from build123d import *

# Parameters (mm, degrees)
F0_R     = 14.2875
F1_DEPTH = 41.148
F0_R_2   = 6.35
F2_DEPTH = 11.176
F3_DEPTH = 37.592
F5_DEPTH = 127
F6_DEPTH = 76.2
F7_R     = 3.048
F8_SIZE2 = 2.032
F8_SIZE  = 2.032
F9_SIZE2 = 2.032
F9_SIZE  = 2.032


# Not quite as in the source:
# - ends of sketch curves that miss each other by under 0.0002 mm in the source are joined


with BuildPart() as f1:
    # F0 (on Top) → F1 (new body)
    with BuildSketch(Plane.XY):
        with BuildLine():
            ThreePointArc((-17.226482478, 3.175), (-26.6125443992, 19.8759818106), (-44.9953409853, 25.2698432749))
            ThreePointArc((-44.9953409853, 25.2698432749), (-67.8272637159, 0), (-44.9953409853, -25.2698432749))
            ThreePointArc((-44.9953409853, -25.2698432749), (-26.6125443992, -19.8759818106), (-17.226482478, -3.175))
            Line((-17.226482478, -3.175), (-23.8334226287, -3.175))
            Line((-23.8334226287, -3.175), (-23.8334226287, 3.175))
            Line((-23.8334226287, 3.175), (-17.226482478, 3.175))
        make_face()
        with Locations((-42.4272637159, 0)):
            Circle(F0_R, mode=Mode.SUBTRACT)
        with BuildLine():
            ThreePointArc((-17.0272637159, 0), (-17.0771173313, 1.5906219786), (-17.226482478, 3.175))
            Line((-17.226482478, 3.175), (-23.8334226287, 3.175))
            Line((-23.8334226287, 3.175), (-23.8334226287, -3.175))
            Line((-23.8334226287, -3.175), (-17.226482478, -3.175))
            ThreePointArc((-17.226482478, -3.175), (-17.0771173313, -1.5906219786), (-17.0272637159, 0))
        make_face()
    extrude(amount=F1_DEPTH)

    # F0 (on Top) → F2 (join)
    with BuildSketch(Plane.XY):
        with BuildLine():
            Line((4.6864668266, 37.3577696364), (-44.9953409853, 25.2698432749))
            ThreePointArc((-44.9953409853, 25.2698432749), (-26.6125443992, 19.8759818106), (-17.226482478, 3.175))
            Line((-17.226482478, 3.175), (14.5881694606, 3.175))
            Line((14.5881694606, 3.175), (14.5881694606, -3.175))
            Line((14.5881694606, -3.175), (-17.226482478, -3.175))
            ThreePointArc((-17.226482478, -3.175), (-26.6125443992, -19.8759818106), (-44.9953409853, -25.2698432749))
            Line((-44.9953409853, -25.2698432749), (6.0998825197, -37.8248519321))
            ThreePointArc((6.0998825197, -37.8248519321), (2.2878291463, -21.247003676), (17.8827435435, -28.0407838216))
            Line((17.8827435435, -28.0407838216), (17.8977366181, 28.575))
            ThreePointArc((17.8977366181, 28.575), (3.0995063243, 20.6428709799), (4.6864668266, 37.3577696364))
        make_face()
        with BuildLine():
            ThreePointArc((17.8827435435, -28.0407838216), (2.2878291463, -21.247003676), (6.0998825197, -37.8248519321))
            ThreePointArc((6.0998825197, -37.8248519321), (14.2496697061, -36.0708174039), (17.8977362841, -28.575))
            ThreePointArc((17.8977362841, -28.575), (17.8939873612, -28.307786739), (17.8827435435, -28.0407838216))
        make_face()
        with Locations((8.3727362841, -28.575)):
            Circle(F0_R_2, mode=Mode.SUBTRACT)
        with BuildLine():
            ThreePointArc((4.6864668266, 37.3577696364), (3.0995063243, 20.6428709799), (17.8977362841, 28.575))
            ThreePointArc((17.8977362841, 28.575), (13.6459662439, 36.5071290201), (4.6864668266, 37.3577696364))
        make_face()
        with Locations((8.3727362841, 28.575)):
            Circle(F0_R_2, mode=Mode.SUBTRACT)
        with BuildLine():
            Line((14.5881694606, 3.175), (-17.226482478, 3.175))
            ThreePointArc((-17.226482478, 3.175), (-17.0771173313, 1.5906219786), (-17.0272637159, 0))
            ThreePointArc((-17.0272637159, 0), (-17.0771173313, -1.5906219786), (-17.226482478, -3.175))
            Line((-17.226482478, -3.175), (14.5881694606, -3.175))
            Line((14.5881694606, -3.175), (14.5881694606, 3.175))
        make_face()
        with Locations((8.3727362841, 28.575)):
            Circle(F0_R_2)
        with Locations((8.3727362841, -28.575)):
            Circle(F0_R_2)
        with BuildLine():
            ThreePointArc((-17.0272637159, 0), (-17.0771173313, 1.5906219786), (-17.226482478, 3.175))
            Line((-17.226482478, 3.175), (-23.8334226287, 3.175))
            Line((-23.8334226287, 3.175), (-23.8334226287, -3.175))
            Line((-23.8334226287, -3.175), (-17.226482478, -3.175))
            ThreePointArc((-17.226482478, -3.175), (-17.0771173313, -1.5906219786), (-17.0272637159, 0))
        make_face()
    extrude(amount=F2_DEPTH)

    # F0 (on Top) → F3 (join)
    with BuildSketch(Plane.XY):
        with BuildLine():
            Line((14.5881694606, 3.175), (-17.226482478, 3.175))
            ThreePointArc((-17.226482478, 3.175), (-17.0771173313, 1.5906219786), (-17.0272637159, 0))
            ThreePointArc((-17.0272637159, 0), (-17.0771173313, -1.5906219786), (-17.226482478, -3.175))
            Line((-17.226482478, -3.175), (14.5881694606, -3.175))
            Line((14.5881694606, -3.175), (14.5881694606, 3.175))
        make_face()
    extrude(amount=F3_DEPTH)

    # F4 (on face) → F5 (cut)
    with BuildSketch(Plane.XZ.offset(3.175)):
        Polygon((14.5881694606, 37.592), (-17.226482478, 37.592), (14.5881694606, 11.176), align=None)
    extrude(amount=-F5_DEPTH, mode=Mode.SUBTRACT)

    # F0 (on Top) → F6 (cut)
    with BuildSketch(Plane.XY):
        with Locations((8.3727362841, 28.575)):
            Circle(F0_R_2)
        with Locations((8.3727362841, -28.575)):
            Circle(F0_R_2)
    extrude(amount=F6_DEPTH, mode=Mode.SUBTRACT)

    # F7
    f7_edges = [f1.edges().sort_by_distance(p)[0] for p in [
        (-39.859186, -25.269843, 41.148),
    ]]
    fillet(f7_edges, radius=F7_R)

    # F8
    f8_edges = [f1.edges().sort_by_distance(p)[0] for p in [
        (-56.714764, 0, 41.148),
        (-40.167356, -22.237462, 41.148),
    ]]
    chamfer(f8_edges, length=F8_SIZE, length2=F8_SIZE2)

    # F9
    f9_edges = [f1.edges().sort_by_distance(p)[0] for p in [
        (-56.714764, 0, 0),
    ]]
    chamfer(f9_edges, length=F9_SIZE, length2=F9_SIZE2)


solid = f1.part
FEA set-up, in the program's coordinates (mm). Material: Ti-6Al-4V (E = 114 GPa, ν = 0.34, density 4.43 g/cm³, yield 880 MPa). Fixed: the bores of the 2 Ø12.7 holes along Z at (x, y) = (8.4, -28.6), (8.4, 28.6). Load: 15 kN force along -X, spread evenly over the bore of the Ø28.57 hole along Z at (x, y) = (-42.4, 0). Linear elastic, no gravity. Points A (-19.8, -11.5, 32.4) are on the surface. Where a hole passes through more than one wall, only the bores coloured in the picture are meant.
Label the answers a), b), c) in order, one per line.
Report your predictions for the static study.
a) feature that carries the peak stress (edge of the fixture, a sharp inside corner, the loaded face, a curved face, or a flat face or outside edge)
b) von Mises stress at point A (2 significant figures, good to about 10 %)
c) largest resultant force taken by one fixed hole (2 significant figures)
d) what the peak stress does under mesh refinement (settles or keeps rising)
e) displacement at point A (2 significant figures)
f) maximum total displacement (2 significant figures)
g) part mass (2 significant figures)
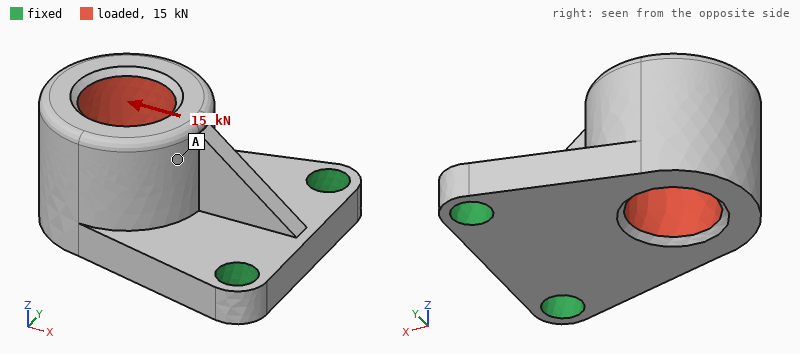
a) edge of the fixture
b) 25 MPa
c) 8.0 kN
d) keeps rising
e) 0.15 mm
f) 0.36 mm
g) 390 g
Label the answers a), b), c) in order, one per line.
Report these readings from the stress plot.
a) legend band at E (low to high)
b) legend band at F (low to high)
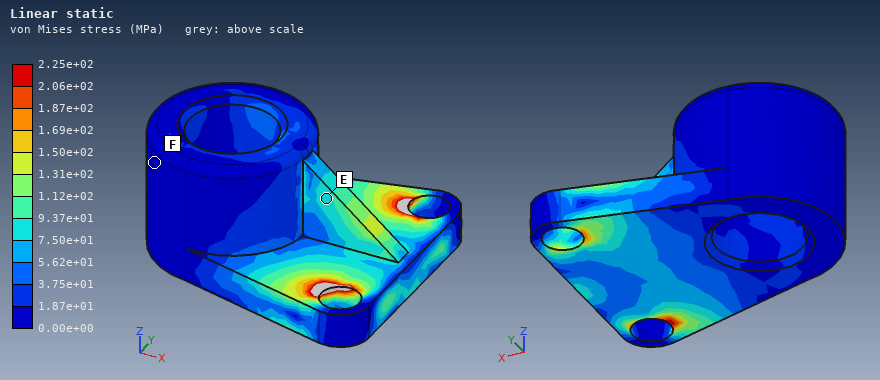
a) 7.50e+01 to 9.37e+01 MPa
b) 0.00e+00 to 1.87e+01 MPa
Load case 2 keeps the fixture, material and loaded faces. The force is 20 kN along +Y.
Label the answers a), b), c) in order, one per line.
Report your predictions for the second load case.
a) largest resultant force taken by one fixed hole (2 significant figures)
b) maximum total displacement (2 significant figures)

a) 20 kN
b) 0.19 mm
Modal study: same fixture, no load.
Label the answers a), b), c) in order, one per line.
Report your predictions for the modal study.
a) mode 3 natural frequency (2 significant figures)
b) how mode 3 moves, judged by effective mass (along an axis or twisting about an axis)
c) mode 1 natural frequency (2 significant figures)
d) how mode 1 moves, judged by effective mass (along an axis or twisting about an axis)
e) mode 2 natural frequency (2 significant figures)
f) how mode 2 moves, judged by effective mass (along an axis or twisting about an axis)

a) 6100 Hz
b) along Y
c) 1400 Hz
d) along Z
e) 3600 Hz
f) along Y
